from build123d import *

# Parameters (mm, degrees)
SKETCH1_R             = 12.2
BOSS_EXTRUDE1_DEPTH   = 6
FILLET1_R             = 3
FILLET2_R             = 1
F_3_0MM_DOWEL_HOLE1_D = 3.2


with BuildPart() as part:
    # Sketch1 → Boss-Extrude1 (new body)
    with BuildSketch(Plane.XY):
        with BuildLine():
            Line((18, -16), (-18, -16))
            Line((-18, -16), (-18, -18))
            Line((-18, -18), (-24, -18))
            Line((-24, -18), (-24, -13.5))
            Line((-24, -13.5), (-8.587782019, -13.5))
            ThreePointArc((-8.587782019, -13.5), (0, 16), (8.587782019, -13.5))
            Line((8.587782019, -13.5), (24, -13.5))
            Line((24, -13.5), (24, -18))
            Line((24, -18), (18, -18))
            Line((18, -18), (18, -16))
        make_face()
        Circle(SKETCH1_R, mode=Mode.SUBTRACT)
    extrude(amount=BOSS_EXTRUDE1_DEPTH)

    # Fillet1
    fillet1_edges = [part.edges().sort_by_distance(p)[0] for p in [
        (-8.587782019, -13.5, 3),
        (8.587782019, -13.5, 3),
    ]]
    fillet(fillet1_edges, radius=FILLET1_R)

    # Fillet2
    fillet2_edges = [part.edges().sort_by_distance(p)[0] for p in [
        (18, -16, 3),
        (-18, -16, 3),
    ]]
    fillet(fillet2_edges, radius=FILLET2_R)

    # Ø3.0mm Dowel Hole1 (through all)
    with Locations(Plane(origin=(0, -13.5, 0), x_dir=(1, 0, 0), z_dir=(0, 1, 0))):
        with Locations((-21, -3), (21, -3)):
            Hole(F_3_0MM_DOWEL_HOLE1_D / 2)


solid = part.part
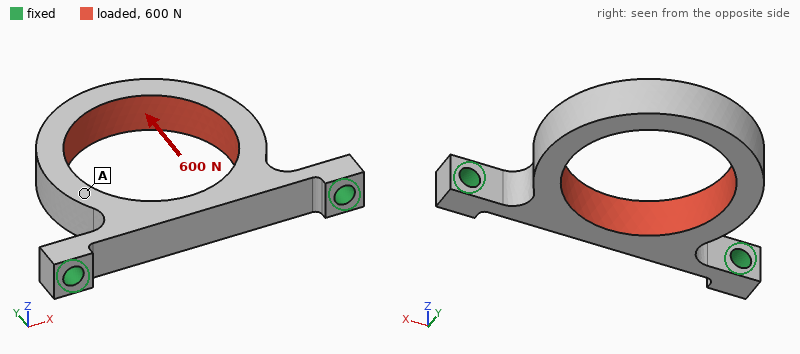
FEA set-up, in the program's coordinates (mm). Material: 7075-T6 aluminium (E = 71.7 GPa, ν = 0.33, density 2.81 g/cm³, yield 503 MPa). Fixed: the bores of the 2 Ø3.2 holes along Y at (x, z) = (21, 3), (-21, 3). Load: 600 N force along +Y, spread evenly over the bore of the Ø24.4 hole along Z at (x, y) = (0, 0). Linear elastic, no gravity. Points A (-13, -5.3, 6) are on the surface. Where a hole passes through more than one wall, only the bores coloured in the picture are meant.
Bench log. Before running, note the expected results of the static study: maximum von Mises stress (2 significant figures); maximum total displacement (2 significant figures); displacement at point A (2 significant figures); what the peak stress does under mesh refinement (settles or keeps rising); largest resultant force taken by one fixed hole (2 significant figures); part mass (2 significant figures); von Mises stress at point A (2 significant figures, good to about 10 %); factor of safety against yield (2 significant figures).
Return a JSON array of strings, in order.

["180 MPa", "31 µm", "22 µm", "settles", "380 N", "7.7 g", "19 MPa", "2.7"]
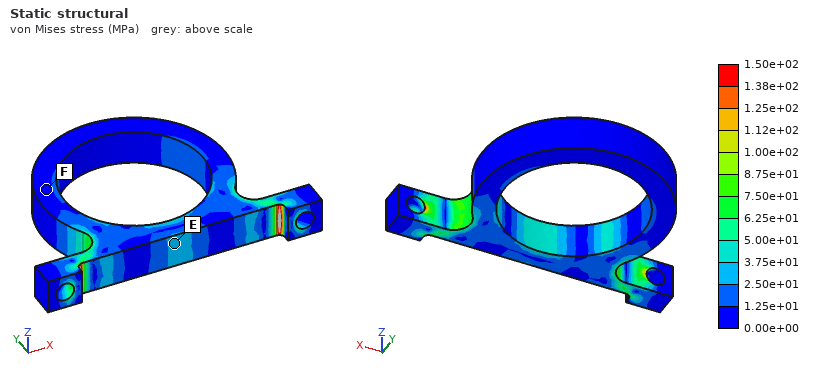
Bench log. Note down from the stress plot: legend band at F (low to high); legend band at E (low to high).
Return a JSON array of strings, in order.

["0.00e+00 to 1.25e+01 MPa", "2.50e+01 to 3.75e+01 MPa"]
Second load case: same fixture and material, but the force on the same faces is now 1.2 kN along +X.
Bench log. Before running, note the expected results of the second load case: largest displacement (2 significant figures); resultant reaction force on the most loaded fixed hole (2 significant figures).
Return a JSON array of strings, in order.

["0.23 mm", "810 N"]
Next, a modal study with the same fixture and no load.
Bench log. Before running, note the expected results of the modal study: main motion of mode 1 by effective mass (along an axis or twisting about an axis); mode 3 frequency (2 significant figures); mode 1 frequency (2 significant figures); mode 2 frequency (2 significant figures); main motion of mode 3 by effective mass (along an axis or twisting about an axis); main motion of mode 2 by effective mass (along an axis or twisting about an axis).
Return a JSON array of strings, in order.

["along Z", "6900 Hz", "1900 Hz", "5200 Hz", "twisting about Y", "along X"]
